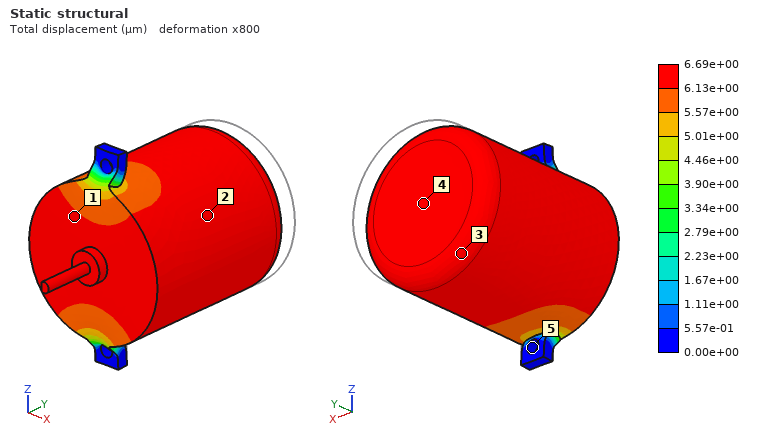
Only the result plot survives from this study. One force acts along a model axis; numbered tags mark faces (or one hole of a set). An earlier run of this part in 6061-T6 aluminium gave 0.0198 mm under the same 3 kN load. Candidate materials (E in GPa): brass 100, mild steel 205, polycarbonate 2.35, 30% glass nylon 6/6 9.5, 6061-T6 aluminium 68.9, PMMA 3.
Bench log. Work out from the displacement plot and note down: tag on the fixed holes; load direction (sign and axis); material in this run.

5
-Y
mild steel
